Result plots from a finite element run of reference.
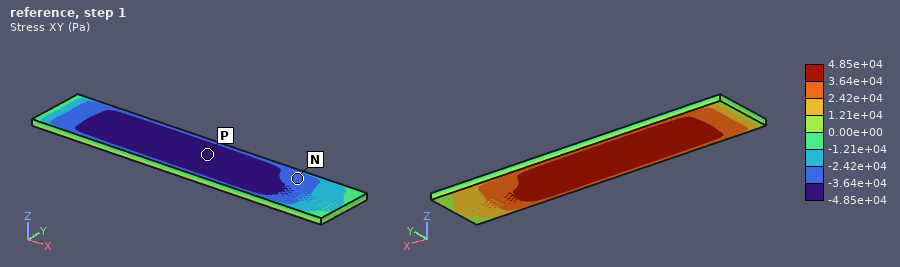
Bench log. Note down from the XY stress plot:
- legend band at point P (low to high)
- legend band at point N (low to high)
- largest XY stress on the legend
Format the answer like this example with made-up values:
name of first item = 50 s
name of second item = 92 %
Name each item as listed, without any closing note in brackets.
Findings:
legend band at point P = -4.85e+04 to -3.64e+04 Pa
legend band at point N = -3.64e+04 to -2.42e+04 Pa
largest XY stress on the legend = 4.85e+04 Pa
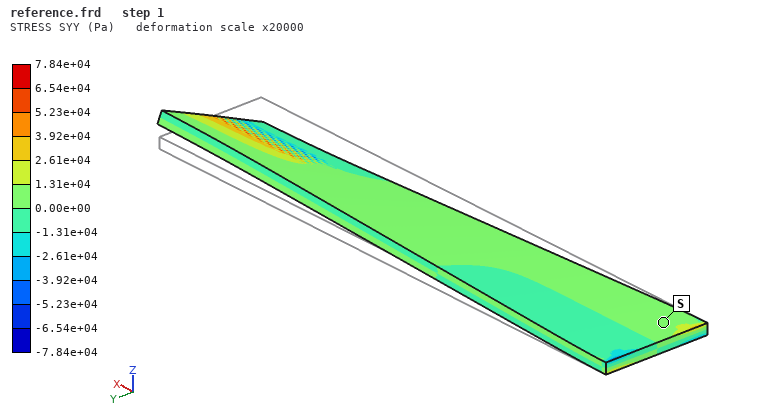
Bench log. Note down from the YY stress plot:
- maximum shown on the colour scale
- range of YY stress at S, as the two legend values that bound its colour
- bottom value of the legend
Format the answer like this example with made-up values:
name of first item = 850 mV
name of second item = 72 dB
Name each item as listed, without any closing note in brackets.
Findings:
maximum shown on the colour scale = 7.84e+04 Pa
range of YY stress at S, as the two legend values that bound its colour = 0.00e+00 to 1.31e+04 Pa
bottom value of the legend = -7.84e+04 Pa
